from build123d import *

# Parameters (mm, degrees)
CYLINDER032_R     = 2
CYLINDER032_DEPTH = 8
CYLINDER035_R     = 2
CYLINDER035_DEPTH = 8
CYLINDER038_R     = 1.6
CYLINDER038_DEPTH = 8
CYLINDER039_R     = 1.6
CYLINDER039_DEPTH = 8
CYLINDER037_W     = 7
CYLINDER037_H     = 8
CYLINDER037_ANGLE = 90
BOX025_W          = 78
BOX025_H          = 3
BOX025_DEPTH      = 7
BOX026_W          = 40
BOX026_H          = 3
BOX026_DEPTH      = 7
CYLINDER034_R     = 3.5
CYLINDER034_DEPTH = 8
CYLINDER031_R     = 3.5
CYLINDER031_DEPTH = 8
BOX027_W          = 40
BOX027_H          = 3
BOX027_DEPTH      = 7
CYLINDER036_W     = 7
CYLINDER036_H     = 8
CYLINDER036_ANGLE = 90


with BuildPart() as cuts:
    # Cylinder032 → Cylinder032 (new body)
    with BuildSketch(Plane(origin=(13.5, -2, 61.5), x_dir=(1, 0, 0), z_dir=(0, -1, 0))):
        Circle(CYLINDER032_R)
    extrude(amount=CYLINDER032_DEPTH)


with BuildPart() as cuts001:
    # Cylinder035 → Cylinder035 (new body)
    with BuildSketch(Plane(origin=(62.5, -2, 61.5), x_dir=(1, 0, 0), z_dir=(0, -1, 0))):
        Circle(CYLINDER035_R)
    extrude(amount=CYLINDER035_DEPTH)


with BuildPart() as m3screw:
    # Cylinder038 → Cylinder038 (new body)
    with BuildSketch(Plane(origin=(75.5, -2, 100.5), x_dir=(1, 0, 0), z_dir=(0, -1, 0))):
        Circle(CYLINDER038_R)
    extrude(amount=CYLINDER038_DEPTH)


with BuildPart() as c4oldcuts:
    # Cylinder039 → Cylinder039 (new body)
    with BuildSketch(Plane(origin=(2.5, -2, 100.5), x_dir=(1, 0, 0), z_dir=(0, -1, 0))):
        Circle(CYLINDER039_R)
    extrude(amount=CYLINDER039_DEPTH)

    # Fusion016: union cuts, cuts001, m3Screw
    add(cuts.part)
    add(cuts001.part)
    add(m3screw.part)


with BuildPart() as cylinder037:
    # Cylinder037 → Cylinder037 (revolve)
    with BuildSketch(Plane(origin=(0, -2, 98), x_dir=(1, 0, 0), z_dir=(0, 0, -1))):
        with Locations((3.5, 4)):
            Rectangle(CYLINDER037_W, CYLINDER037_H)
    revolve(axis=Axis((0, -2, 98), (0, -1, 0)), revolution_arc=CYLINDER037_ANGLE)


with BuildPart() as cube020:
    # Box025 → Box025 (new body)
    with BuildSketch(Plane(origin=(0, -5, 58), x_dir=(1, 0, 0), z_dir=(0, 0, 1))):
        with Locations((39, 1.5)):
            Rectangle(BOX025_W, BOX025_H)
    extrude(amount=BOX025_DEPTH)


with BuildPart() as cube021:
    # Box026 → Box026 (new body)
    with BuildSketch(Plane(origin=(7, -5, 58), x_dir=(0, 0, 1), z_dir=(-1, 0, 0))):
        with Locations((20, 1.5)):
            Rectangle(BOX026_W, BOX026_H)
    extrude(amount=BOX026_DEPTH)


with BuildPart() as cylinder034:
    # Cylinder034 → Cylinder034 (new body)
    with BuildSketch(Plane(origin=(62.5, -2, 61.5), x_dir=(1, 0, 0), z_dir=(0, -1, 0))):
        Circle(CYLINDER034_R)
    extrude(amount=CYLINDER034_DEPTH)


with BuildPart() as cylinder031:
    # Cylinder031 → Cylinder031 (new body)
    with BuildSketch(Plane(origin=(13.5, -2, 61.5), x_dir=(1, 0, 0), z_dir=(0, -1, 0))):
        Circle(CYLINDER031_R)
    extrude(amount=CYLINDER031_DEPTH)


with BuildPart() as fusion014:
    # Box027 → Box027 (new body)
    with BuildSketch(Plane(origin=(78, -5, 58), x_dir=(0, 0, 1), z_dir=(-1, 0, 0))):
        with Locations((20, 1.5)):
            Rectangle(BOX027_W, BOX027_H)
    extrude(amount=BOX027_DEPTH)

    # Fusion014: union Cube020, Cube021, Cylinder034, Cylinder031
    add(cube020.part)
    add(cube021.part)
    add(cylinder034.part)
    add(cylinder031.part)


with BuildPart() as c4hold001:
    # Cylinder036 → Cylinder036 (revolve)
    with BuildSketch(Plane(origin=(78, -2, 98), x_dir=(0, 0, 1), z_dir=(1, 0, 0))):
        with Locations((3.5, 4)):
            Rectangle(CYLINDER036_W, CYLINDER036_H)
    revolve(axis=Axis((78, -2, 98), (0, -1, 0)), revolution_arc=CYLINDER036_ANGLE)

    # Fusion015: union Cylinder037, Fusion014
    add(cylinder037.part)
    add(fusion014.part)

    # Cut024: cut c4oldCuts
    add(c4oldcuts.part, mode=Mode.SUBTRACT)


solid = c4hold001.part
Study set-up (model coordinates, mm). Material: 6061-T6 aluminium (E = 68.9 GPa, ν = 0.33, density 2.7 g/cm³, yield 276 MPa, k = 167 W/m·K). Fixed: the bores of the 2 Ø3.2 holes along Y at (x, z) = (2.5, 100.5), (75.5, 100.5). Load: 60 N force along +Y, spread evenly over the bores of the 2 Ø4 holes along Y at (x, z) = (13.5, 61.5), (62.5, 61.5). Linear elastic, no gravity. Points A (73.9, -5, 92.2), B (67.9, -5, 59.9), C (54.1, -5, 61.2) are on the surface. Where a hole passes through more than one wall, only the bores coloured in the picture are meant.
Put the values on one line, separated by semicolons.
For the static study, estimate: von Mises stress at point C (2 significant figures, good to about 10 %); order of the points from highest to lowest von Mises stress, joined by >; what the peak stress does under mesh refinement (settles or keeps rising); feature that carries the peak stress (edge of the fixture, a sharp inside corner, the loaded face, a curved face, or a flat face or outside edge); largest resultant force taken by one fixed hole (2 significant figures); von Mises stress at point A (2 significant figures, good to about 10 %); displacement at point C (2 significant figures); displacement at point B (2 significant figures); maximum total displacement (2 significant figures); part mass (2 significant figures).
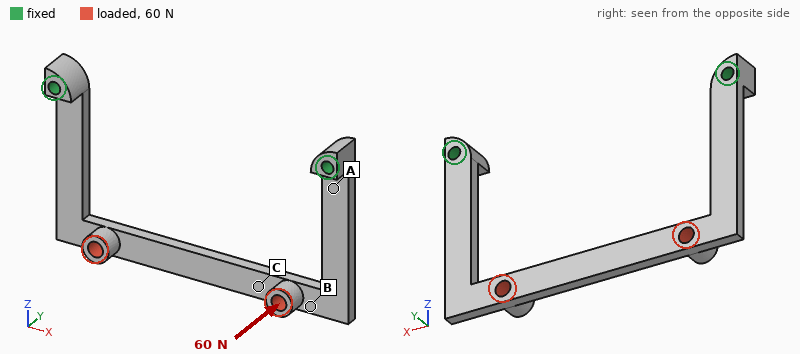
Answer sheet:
18 MPa; A > C > B; keeps rising; edge of the fixture; 31 N; 88 MPa; 0.57 mm; 0.55 mm; 0.66 mm; 10.0 g
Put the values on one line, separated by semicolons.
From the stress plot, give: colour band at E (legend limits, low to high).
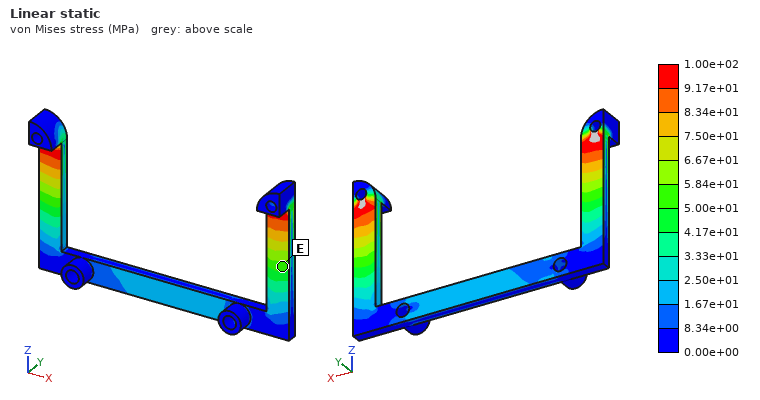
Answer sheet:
5.00e+01 to 5.84e+01 MPa
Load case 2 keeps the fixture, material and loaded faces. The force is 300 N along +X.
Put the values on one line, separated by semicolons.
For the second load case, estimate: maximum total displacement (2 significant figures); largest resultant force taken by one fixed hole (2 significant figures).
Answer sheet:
0.25 mm; 160 N
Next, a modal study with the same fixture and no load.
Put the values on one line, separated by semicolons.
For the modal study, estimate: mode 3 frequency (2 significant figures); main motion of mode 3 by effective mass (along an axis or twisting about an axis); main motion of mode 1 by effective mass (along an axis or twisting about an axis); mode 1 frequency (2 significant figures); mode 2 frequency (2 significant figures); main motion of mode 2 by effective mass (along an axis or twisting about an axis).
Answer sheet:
2400 Hz; along X; along Y; 700 Hz; 1400 Hz; twisting about Z
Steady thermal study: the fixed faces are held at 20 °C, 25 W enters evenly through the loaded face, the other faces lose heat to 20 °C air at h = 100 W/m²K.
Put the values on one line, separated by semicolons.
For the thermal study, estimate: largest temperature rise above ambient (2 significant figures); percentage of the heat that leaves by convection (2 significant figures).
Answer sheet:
80 K; 61 %
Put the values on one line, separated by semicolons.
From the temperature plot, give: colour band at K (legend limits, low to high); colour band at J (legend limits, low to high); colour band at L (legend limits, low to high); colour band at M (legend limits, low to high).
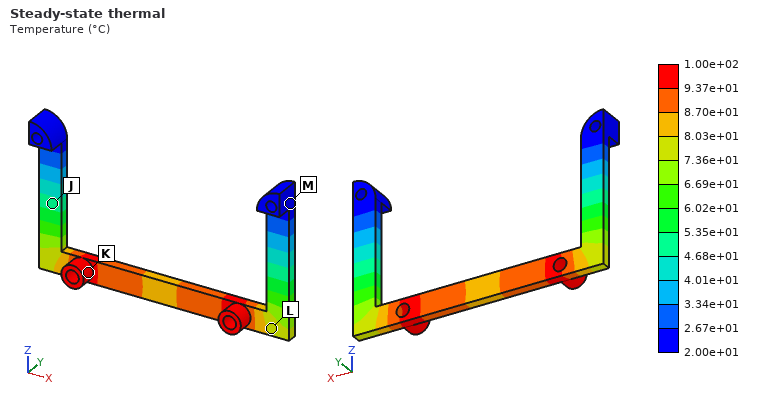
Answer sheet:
9.37e+01 to 1.00e+02 °C; 4.68e+01 to 5.35e+01 °C; 7.36e+01 to 8.03e+01 °C; 2.00e+01 to 2.67e+01 °C
